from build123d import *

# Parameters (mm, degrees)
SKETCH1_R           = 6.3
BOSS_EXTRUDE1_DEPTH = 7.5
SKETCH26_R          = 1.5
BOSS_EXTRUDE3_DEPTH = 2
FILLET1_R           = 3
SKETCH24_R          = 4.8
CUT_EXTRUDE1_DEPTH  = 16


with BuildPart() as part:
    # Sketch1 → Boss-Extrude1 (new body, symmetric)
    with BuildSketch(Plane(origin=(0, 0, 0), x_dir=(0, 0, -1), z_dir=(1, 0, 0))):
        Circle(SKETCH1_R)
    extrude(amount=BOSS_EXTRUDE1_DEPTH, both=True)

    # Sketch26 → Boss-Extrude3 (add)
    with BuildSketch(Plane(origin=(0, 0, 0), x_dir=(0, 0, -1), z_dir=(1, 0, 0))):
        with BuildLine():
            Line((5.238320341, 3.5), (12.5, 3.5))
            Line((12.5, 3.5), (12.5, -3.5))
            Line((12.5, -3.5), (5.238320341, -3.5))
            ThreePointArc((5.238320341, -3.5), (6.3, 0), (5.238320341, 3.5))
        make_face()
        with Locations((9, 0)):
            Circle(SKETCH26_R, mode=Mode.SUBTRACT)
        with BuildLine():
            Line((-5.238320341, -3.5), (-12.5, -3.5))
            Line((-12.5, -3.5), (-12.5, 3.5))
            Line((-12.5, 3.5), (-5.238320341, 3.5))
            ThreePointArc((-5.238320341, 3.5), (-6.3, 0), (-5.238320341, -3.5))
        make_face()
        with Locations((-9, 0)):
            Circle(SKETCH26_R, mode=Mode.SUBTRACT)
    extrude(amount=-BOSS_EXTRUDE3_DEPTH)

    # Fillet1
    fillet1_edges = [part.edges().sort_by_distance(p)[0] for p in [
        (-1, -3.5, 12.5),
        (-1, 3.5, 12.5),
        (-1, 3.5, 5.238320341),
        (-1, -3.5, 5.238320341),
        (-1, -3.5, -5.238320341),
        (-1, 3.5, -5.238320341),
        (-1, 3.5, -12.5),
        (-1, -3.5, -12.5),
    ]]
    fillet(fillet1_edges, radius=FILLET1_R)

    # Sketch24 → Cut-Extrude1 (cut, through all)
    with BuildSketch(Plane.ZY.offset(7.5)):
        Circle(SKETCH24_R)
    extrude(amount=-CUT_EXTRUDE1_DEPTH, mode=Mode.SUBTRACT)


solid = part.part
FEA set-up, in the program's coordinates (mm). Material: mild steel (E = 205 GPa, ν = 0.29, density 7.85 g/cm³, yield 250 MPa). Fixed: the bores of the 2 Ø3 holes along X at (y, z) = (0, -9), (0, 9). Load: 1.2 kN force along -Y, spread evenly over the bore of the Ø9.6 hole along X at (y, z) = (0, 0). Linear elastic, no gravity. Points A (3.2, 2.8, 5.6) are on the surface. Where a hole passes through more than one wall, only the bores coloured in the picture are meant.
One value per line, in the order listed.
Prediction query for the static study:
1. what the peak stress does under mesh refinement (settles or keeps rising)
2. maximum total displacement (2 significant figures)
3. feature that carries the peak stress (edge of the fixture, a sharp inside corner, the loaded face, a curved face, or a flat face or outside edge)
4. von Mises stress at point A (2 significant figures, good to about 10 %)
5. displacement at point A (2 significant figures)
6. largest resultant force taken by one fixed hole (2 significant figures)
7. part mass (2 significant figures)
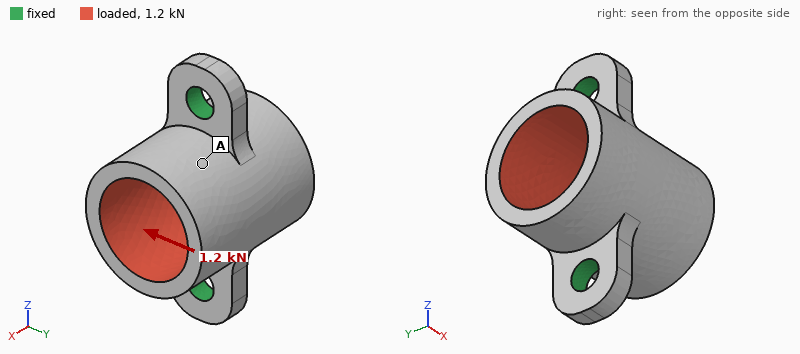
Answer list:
keeps rising
13 µm
edge of the fixture
20 MPa
6.8 µm
600 N
7.3 g
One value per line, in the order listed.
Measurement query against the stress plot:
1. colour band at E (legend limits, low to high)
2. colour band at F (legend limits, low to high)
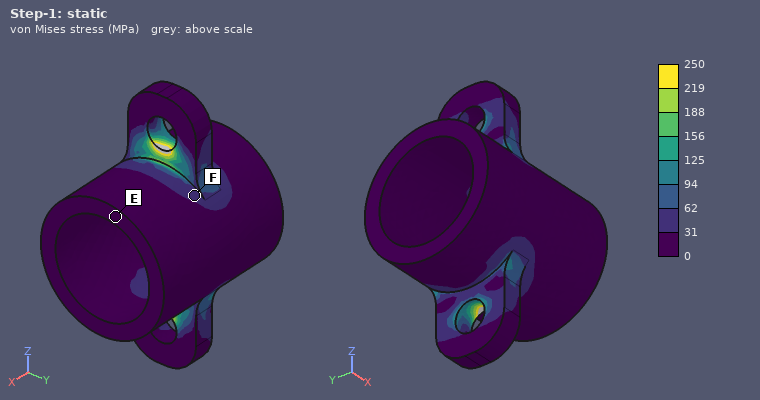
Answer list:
0 to 31 MPa
31 to 62 MPa
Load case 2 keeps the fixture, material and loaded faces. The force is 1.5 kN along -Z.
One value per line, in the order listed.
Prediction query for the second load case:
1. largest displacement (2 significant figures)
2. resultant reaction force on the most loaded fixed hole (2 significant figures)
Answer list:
4.3 µm
760 N
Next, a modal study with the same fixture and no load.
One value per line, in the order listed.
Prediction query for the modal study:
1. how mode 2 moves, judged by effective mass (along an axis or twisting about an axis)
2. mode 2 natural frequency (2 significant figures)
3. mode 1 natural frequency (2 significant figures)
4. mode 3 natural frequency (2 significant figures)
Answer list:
along X
28 kHz
13 kHz
39 kHz
